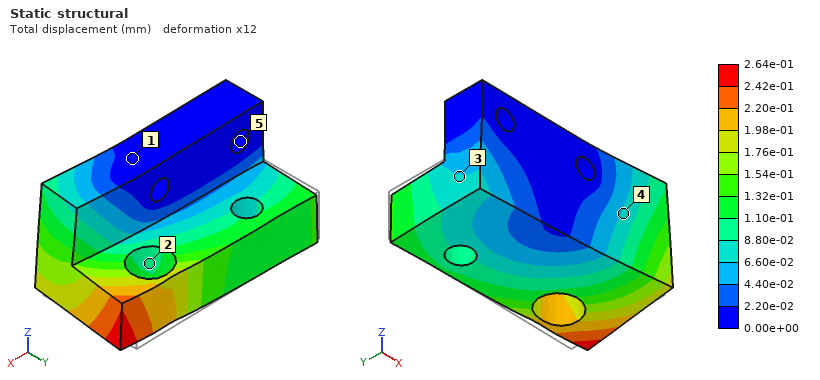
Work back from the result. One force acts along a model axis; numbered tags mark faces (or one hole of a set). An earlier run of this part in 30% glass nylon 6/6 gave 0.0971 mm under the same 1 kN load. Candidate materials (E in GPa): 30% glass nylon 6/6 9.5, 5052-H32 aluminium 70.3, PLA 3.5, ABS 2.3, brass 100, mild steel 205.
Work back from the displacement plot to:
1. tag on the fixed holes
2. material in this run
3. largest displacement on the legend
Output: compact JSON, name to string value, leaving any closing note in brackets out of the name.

{"tag on the fixed holes": "5", "material in this run": "PLA", "largest displacement on the legend": "2.64e-01 mm"}
